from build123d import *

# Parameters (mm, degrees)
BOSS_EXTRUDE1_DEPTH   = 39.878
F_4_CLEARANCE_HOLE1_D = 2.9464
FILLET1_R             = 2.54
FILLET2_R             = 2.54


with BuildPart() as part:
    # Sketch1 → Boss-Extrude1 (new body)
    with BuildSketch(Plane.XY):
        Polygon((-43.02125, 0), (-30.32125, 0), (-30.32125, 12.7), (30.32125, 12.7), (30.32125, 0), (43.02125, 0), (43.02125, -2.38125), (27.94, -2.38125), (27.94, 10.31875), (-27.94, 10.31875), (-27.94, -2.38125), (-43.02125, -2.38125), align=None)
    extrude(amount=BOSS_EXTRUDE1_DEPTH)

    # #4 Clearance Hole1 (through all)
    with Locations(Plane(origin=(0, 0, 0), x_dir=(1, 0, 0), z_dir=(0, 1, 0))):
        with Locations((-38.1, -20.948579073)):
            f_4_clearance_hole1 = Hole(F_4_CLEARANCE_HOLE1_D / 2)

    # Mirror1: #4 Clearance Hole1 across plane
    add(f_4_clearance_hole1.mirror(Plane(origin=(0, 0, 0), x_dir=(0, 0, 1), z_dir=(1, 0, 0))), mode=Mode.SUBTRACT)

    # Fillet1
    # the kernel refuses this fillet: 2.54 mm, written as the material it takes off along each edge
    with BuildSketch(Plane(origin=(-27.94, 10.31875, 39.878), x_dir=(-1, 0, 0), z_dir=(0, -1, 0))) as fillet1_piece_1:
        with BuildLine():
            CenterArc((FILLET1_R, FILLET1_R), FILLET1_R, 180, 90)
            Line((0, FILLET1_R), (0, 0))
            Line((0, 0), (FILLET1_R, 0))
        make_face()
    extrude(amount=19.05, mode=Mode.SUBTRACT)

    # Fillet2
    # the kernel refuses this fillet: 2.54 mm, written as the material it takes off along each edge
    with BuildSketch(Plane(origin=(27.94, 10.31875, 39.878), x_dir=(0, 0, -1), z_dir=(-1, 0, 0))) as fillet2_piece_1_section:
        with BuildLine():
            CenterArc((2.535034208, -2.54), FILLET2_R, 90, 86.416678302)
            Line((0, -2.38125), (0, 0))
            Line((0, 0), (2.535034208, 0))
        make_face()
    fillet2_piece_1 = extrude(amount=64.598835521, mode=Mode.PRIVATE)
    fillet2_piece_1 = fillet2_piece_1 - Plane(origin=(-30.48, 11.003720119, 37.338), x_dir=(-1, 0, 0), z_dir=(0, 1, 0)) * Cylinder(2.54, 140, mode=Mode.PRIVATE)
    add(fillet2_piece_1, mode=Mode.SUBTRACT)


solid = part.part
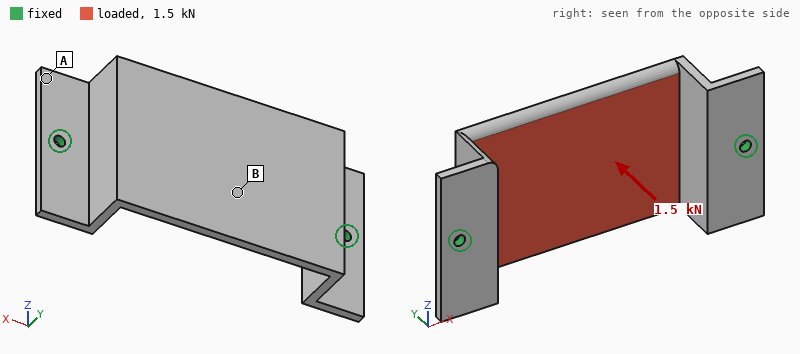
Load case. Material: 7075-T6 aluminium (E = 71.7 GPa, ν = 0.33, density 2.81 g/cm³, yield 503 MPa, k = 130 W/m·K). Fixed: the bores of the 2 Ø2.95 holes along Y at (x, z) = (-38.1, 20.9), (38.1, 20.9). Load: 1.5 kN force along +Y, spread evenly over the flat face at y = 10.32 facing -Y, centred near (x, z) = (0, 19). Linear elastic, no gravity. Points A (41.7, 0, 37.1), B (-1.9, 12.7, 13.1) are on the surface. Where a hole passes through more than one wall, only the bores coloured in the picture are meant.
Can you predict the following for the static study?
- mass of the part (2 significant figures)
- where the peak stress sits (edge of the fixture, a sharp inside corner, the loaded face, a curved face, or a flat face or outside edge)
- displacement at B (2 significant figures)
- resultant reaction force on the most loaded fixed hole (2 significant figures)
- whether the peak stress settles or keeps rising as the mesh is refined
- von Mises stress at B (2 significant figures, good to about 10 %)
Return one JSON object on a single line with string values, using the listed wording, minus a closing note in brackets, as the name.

{"mass of the part": "29 g", "where the peak stress sits": "edge of the fixture", "displacement at B": "0.40 mm", "resultant reaction force on the most loaded fixed hole": "1.1 kN", "whether the peak stress settles or keeps rising as the mesh is refined": "keeps rising", "von Mises stress at B": "120 MPa"}
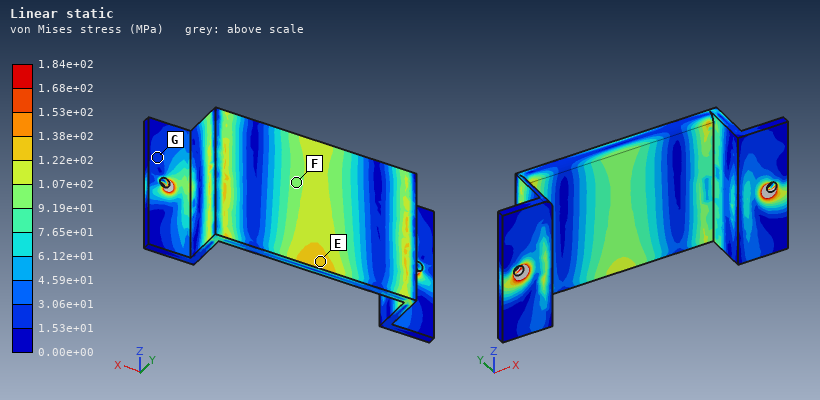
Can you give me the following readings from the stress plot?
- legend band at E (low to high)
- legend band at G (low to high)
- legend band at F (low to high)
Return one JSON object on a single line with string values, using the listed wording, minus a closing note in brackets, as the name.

{"legend band at E": "1.22e+02 to 1.38e+02 MPa", "legend band at G": "1.53e+01 to 3.06e+01 MPa", "legend band at F": "9.19e+01 to 1.07e+02 MPa"}
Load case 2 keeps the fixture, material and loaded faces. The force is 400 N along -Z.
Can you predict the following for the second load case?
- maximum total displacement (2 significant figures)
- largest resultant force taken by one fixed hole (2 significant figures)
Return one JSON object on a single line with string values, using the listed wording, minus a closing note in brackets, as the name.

{"maximum total displacement": "0.17 mm", "largest resultant force taken by one fixed hole": "200 N"}
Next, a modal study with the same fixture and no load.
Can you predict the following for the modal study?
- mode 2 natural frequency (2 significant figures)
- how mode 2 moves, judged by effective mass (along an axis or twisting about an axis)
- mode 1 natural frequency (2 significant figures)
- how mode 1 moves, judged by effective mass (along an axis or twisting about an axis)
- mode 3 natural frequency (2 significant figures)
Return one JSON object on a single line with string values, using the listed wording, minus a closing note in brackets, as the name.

{"mode 2 natural frequency": "2800 Hz", "how mode 2 moves, judged by effective mass": "along X", "mode 1 natural frequency": "1600 Hz", "how mode 1 moves, judged by effective mass": "along Z", "mode 3 natural frequency": "3000 Hz"}
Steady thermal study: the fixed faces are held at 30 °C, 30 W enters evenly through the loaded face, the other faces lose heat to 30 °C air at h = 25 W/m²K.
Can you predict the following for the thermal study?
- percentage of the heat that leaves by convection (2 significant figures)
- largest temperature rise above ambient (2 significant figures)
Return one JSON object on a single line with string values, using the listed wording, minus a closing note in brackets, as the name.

{"percentage of the heat that leaves by convection": "17 %", "largest temperature rise above ambient": "49 K"}
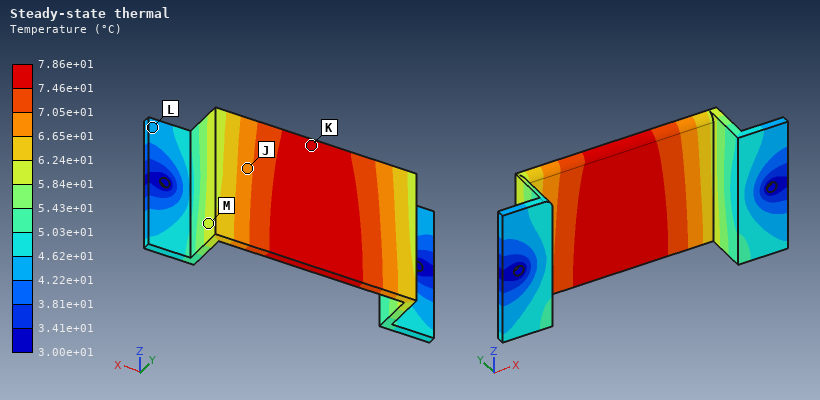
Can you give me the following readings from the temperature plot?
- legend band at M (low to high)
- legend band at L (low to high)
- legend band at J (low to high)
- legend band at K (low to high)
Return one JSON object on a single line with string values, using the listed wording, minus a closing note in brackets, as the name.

{"legend band at M": "5.84e+01 to 6.24e+01 °C", "legend band at L": "4.22e+01 to 4.62e+01 °C", "legend band at J": "6.65e+01 to 7.05e+01 °C", "legend band at K": "7.46e+01 to 7.86e+01 °C"}
